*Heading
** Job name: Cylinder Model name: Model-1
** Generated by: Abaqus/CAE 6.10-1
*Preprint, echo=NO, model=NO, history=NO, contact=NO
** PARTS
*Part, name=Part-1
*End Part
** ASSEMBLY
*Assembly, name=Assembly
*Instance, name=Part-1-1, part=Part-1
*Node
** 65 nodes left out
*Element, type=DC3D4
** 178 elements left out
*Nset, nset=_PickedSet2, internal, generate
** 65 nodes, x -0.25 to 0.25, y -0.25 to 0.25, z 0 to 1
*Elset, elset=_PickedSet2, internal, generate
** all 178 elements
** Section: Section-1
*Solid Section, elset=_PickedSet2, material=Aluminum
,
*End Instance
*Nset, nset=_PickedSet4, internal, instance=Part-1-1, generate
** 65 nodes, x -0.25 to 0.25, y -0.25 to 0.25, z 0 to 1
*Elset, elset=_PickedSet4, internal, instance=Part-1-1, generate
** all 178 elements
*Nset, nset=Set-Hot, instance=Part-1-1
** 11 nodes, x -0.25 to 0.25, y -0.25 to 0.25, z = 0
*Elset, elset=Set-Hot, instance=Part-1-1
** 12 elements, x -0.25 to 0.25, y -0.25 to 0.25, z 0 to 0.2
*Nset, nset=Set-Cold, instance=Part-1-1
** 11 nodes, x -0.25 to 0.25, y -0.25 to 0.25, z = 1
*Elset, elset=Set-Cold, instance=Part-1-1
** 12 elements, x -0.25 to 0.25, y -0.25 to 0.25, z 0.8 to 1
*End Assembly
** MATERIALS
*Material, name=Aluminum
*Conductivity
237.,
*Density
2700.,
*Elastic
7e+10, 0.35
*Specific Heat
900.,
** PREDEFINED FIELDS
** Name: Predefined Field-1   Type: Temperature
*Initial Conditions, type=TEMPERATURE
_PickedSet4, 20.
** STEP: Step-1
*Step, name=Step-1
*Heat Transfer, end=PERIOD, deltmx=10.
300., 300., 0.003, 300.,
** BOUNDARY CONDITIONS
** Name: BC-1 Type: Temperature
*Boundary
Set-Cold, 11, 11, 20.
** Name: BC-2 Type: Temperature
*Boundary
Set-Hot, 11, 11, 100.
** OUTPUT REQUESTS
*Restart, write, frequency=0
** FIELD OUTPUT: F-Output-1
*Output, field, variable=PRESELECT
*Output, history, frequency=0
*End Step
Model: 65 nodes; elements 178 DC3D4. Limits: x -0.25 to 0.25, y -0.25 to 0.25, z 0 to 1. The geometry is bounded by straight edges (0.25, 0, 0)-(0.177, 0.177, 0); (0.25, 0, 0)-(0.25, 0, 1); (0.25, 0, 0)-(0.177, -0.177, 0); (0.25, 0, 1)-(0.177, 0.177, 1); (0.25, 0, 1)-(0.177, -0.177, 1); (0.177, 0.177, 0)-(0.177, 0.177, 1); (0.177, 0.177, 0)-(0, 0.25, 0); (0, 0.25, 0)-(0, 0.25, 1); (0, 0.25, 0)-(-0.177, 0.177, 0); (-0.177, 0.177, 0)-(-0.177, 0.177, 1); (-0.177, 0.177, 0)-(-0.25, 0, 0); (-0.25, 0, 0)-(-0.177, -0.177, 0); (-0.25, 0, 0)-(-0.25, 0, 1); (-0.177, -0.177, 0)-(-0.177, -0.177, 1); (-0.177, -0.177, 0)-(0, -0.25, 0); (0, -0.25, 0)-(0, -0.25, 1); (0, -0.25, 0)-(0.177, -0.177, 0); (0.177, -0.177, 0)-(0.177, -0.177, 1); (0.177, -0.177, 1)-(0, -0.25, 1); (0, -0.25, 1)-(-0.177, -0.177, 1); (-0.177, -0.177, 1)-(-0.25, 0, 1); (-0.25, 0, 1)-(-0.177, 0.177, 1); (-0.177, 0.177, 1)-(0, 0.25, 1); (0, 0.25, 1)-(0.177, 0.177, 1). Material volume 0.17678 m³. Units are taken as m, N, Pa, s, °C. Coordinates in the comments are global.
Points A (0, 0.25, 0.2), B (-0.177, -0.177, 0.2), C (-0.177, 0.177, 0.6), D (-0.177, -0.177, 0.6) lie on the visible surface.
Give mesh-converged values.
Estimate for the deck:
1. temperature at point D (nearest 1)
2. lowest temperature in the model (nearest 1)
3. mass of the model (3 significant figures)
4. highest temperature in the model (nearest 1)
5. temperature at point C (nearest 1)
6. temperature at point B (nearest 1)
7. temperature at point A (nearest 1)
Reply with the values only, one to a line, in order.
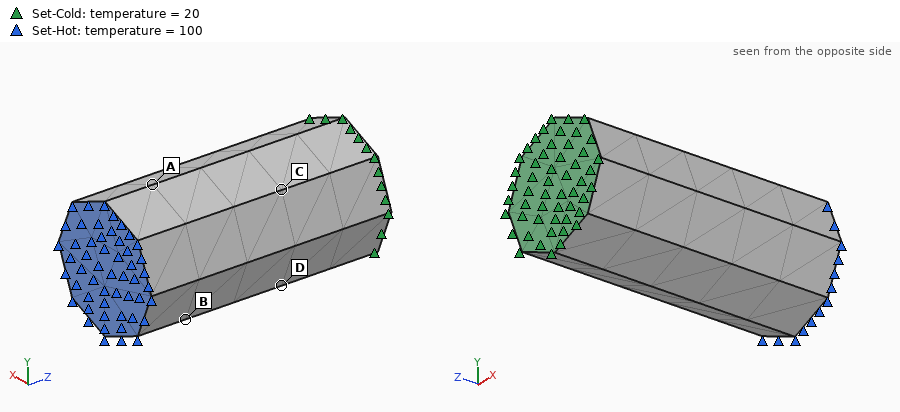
21 °C
20 °C
477 kg
100 °C
21 °C
52 °C
52 °C
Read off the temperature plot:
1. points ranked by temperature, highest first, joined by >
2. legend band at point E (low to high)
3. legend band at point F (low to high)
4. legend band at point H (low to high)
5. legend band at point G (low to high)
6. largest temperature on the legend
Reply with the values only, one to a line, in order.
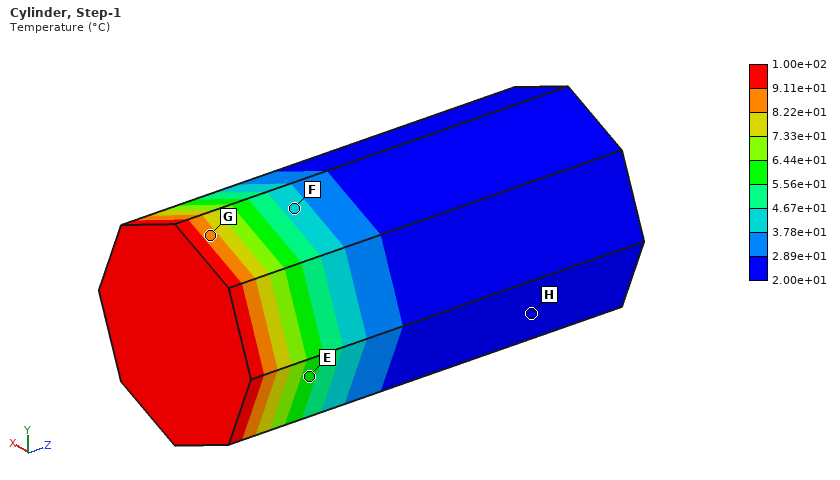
G > E > F > H
5.56e+01 to 6.44e+01 °C
3.78e+01 to 4.67e+01 °C
2.00e+01 to 2.89e+01 °C
8.22e+01 to 9.11e+01 °C
1.00e+02 °C
